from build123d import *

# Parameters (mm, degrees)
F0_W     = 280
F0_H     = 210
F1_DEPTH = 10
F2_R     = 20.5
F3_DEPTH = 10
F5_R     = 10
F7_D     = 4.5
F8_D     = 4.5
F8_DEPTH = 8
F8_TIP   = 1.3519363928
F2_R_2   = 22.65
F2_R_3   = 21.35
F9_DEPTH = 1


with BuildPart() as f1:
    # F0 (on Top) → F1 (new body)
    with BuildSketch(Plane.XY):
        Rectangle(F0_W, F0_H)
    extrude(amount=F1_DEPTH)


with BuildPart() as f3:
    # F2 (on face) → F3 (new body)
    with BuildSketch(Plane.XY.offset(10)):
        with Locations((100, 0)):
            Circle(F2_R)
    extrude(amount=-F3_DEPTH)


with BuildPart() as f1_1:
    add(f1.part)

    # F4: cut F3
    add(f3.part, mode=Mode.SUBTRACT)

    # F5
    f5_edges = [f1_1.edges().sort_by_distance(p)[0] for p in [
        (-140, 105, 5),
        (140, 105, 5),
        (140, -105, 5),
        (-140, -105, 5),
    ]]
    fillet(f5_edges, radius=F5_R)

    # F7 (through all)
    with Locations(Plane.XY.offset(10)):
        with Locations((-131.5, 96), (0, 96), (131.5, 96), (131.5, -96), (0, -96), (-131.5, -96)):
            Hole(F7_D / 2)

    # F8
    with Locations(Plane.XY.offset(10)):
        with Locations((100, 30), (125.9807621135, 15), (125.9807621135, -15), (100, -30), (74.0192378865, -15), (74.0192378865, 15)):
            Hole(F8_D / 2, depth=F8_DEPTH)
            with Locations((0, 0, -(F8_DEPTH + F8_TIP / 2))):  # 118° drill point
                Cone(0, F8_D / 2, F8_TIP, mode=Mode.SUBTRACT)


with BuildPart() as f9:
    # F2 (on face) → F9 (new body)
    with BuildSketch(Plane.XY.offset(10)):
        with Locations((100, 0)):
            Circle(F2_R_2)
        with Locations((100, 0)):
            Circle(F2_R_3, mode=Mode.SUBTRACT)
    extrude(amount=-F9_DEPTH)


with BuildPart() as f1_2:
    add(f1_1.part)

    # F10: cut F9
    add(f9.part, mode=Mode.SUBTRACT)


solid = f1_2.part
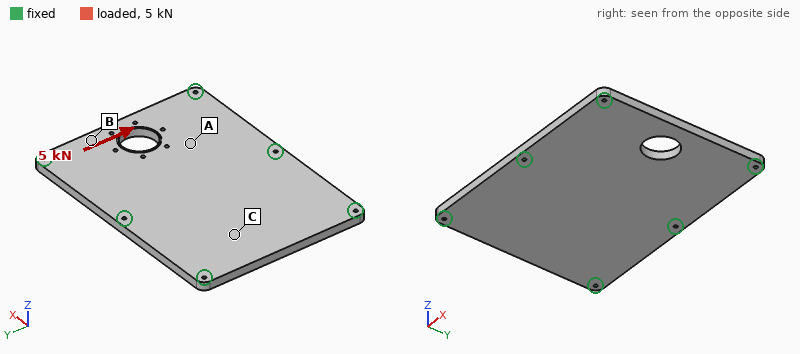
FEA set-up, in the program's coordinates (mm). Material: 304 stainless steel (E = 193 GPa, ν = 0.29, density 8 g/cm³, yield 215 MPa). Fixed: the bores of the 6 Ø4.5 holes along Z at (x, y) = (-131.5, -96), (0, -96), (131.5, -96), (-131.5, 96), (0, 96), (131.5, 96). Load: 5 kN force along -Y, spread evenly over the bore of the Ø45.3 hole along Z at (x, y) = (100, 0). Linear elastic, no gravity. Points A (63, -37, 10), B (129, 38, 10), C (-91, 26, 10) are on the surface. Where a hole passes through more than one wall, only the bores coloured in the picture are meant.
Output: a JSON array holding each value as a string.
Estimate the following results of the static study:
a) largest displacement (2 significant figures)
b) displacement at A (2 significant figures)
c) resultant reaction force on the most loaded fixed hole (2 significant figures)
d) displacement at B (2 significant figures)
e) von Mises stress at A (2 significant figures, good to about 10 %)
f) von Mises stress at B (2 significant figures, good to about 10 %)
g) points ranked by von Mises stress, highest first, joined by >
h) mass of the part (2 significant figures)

["3.5 µm", "2.4 µm", "1.6 kN", "3.2 µm", "3.2 MPa", "6.9 MPa", "B > A > C", "4.6 kg"]
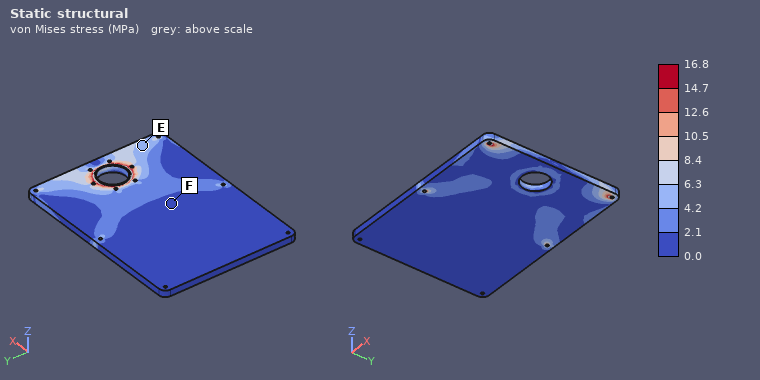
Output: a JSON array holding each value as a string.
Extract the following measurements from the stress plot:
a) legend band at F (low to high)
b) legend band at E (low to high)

["0.0 to 2.1 MPa", "4.2 to 6.3 MPa"]
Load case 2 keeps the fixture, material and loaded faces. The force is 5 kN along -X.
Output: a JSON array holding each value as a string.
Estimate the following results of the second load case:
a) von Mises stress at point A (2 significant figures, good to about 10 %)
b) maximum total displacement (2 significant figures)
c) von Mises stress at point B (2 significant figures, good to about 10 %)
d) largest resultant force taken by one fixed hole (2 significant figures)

["6.4 MPa", "15 µm", "7.0 MPa", "1.3 kN"]
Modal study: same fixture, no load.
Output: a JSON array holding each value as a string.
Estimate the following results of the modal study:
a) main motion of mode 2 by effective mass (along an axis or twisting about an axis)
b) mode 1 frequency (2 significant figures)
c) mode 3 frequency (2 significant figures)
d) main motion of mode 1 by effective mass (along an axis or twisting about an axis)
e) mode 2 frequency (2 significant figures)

["twisting about Y", "930 Hz", "1800 Hz", "along Z", "1100 Hz"]
